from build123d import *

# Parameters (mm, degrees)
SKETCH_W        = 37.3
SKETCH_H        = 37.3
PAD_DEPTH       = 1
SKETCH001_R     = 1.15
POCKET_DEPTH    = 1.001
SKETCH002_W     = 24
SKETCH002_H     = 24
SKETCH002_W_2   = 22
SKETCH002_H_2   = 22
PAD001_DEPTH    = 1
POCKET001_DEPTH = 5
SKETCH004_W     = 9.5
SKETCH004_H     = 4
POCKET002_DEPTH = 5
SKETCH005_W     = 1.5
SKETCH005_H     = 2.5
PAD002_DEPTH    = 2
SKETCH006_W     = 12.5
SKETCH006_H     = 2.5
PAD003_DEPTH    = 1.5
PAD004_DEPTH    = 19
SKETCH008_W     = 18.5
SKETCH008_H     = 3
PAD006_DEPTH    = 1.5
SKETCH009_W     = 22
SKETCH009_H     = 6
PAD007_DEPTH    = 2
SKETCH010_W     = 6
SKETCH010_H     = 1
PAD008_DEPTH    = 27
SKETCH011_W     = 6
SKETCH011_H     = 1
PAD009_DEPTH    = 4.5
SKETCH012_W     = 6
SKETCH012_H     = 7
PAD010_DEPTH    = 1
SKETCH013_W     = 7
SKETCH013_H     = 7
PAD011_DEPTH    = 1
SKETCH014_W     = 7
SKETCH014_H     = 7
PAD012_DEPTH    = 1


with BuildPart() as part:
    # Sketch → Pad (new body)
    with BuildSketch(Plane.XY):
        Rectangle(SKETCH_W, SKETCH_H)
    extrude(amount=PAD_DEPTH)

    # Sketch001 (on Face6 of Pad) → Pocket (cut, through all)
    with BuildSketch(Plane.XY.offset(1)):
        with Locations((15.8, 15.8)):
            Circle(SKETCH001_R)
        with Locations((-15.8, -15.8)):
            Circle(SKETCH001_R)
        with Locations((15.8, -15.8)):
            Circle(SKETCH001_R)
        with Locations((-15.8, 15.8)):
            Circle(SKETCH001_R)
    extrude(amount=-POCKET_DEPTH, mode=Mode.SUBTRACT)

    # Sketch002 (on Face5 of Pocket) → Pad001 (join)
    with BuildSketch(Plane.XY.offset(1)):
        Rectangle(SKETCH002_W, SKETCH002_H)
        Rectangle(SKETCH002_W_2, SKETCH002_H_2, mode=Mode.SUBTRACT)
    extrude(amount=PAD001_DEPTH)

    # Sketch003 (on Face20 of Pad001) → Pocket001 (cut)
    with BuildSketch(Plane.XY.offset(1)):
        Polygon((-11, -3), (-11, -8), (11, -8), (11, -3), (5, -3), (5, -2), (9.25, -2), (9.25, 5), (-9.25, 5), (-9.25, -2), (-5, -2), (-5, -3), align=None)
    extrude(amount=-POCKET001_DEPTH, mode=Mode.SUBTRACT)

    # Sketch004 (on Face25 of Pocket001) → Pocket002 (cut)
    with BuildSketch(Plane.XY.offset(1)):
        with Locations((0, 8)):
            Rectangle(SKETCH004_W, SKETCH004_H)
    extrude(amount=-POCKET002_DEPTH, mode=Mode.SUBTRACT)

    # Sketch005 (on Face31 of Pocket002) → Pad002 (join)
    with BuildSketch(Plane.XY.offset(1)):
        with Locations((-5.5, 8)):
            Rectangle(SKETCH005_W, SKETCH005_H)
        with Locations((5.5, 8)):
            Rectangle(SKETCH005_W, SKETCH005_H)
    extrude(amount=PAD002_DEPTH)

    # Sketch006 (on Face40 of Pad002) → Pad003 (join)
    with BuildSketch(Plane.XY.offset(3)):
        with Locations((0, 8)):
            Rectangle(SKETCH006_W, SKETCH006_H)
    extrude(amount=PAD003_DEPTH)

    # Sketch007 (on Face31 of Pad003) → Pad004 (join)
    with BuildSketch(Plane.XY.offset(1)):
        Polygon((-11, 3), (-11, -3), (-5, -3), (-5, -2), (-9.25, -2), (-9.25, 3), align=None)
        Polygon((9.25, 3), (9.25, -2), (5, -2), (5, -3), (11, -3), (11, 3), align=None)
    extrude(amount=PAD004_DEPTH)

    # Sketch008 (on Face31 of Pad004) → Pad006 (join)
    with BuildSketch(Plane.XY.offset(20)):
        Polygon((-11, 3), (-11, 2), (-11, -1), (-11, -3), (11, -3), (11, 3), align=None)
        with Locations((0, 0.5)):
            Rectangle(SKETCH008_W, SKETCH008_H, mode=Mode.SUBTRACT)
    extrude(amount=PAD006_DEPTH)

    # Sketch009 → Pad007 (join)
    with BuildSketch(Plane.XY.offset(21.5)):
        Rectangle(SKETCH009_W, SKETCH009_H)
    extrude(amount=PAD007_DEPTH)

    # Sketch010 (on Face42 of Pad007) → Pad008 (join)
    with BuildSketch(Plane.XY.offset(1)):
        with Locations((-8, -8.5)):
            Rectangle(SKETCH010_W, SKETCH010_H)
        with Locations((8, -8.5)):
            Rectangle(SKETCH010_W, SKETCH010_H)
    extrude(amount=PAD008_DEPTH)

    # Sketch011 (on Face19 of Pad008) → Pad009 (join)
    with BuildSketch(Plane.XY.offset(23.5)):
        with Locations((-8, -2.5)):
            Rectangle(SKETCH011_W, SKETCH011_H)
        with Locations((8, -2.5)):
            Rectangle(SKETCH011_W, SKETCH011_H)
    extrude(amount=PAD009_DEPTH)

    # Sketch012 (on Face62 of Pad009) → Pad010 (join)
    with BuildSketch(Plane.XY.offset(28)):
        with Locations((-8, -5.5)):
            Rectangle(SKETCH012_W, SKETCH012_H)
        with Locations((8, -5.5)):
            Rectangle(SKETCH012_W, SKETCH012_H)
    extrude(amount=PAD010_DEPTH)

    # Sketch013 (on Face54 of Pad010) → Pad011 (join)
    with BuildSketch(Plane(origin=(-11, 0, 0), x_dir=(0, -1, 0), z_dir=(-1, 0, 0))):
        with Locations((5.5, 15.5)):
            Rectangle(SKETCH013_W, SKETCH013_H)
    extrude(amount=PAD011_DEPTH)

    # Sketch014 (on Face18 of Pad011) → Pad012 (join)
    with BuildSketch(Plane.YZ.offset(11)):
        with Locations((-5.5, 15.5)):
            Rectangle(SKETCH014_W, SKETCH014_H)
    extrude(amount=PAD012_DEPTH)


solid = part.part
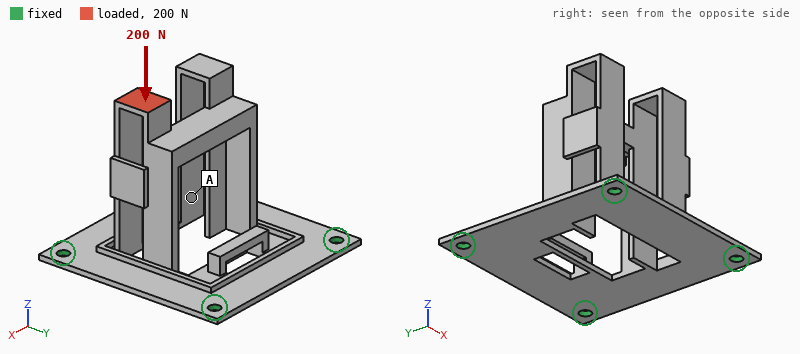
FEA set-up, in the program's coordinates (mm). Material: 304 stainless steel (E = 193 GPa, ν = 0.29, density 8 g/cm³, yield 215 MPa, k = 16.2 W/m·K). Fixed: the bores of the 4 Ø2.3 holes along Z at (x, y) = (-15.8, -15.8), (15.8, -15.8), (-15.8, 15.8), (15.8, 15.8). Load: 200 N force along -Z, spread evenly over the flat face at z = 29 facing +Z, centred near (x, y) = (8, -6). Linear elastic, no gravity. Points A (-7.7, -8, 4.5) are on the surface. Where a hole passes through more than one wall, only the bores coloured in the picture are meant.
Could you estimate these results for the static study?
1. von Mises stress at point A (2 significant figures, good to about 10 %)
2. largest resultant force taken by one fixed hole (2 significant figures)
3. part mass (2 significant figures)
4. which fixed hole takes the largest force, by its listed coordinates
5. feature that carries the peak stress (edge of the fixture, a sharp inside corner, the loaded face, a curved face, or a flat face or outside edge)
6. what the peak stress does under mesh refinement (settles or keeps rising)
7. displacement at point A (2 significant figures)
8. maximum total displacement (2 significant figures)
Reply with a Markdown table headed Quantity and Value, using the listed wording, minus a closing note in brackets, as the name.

| Quantity | Value |
|---|---|
| von Mises stress at point A | 21 MPa |
| largest resultant force taken by one fixed hole | 130 N |
| part mass | 22 g |
| which fixed hole takes the largest force, by its listed coordinates | (15.8, -15.8) |
| feature that carries the peak stress | edge of the fixture |
| what the peak stress does under mesh refinement | keeps rising |
| displacement at point A | 21 µm |
| maximum total displacement | 57 µm |
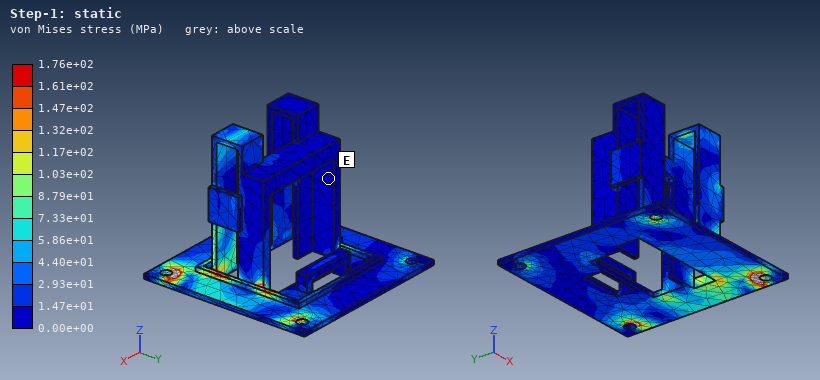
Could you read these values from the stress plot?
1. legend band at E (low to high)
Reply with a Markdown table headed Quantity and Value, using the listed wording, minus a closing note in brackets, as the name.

| Quantity | Value |
|---|---|
| legend band at E | 0.00e+00 to 1.47e+01 MPa |
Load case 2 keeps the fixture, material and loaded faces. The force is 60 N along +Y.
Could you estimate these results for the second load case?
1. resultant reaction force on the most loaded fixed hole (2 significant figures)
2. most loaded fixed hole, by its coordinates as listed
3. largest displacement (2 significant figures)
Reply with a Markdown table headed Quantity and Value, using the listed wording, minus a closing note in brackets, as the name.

| Quantity | Value |
|---|---|
| resultant reaction force on the most loaded fixed hole | 52 N |
| most loaded fixed hole, by its coordinates as listed | (15.8, 15.8) |
| largest displacement | 0.11 mm |
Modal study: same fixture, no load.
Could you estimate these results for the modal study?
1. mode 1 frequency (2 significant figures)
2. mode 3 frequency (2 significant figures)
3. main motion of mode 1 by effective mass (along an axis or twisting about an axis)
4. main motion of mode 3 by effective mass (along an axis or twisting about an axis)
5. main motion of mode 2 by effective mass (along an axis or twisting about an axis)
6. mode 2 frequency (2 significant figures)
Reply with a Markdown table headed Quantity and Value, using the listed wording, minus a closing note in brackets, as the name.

| Quantity | Value |
|---|---|
| mode 1 frequency | 2000 Hz |
| mode 3 frequency | 3200 Hz |
| main motion of mode 1 by effective mass | along Y |
| main motion of mode 3 by effective mass | along Z |
| main motion of mode 2 by effective mass | along X |
| mode 2 frequency | 2300 Hz |
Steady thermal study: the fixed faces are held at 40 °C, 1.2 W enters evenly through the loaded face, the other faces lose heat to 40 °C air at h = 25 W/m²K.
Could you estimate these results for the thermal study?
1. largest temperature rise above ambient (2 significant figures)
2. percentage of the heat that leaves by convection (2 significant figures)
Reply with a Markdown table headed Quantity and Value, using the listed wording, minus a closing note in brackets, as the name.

| Quantity | Value |
|---|---|
| largest temperature rise above ambient | 69 K |
| percentage of the heat that leaves by convection | 85 % |
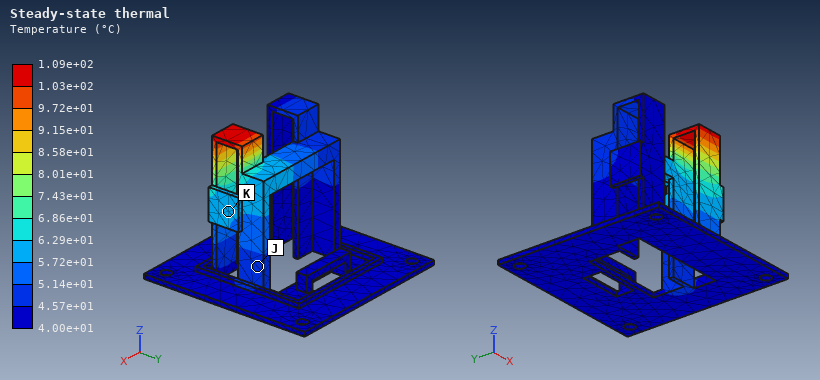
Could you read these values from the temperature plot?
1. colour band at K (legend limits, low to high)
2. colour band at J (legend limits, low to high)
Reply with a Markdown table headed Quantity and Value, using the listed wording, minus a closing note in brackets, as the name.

| Quantity | Value |
|---|---|
| colour band at K | 5.72e+01 to 6.29e+01 °C |
| colour band at J | 4.57e+01 to 5.14e+01 °C |
